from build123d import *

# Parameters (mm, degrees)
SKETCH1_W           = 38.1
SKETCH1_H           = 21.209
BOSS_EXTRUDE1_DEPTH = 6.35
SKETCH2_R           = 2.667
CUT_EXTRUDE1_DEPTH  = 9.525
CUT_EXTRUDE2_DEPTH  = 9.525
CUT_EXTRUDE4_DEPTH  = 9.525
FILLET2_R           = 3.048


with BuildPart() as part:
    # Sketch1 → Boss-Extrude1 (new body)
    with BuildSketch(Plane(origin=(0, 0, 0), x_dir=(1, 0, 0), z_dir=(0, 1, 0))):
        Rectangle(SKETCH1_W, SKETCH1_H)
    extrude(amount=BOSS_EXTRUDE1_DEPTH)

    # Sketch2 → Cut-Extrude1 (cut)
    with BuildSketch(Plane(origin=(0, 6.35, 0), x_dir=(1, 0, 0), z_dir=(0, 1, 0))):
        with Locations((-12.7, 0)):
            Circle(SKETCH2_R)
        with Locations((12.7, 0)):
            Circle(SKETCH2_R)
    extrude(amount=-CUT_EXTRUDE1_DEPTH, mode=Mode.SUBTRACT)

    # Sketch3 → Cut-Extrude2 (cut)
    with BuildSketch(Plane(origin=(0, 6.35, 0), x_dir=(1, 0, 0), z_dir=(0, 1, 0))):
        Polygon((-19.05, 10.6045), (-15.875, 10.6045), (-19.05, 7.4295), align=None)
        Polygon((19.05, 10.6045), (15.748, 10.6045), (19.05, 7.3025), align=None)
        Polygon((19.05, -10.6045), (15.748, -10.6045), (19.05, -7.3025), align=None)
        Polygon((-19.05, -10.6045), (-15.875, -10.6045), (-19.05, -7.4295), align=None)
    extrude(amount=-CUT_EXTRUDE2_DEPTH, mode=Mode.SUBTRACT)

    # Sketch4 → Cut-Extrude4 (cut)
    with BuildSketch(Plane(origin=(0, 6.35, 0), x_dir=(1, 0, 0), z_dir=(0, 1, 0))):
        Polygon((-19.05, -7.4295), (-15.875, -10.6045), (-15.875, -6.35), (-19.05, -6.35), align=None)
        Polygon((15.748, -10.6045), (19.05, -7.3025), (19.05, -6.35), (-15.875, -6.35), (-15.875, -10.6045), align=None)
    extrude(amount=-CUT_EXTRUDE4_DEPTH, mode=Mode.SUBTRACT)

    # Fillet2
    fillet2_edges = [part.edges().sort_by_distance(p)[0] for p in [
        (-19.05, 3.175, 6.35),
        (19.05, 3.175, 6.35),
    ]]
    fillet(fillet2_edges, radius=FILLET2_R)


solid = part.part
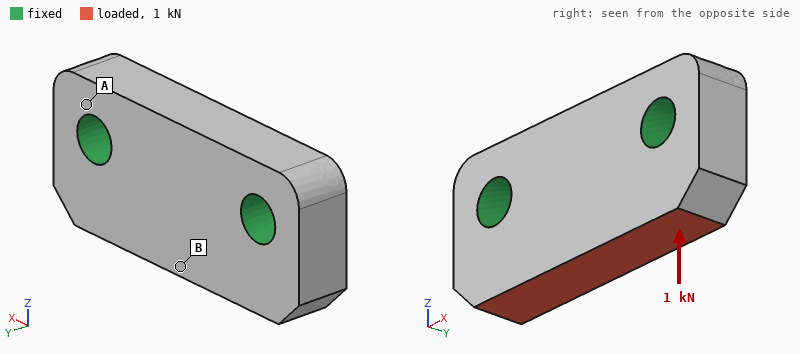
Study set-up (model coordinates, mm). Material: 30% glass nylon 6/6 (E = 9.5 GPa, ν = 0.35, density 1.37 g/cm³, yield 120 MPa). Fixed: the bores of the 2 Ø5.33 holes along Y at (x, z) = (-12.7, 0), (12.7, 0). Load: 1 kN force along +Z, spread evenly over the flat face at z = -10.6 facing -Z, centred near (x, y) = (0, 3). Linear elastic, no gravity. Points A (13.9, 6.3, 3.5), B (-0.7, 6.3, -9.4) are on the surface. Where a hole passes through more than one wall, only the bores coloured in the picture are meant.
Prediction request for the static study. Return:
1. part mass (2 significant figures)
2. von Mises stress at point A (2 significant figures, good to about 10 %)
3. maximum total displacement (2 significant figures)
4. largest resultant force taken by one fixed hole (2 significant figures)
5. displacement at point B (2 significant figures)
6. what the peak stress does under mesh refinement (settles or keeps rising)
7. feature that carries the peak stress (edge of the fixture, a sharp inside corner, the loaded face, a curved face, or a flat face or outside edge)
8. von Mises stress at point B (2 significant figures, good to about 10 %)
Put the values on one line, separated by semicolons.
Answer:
5.1 g; 1.9 MPa; 11 µm; 520 N; 11 µm; keeps rising; edge of the fixture; 5.0 MPa
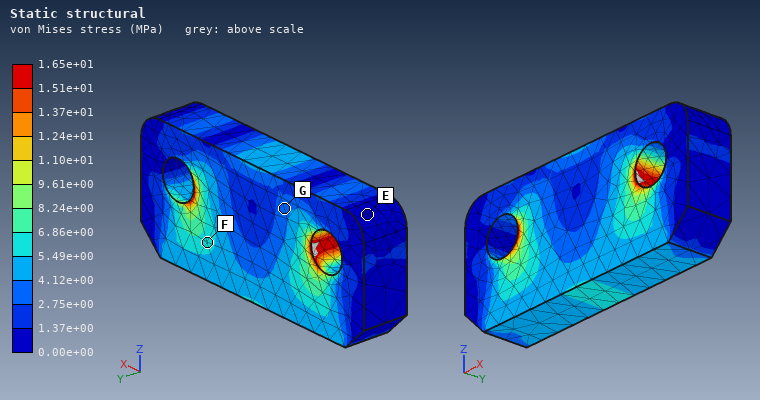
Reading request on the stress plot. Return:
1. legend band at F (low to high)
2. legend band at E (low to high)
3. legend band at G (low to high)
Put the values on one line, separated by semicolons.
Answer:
5.49e+00 to 6.86e+00 MPa; 0.00e+00 to 1.37e+00 MPa; 2.75e+00 to 4.12e+00 MPa
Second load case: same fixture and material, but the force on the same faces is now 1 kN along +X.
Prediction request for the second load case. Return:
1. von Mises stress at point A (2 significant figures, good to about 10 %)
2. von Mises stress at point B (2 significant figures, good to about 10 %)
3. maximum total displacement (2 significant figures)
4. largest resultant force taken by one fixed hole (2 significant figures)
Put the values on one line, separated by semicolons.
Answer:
2.0 MPa; 9.0 MPa; 18 µm; 600 N
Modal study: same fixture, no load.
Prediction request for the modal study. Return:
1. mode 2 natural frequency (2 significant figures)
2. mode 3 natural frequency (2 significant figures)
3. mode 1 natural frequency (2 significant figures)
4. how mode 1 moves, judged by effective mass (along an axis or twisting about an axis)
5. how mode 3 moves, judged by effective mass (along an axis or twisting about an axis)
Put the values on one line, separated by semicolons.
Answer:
24 kHz; 27 kHz; 17 kHz; along Y; along Z
